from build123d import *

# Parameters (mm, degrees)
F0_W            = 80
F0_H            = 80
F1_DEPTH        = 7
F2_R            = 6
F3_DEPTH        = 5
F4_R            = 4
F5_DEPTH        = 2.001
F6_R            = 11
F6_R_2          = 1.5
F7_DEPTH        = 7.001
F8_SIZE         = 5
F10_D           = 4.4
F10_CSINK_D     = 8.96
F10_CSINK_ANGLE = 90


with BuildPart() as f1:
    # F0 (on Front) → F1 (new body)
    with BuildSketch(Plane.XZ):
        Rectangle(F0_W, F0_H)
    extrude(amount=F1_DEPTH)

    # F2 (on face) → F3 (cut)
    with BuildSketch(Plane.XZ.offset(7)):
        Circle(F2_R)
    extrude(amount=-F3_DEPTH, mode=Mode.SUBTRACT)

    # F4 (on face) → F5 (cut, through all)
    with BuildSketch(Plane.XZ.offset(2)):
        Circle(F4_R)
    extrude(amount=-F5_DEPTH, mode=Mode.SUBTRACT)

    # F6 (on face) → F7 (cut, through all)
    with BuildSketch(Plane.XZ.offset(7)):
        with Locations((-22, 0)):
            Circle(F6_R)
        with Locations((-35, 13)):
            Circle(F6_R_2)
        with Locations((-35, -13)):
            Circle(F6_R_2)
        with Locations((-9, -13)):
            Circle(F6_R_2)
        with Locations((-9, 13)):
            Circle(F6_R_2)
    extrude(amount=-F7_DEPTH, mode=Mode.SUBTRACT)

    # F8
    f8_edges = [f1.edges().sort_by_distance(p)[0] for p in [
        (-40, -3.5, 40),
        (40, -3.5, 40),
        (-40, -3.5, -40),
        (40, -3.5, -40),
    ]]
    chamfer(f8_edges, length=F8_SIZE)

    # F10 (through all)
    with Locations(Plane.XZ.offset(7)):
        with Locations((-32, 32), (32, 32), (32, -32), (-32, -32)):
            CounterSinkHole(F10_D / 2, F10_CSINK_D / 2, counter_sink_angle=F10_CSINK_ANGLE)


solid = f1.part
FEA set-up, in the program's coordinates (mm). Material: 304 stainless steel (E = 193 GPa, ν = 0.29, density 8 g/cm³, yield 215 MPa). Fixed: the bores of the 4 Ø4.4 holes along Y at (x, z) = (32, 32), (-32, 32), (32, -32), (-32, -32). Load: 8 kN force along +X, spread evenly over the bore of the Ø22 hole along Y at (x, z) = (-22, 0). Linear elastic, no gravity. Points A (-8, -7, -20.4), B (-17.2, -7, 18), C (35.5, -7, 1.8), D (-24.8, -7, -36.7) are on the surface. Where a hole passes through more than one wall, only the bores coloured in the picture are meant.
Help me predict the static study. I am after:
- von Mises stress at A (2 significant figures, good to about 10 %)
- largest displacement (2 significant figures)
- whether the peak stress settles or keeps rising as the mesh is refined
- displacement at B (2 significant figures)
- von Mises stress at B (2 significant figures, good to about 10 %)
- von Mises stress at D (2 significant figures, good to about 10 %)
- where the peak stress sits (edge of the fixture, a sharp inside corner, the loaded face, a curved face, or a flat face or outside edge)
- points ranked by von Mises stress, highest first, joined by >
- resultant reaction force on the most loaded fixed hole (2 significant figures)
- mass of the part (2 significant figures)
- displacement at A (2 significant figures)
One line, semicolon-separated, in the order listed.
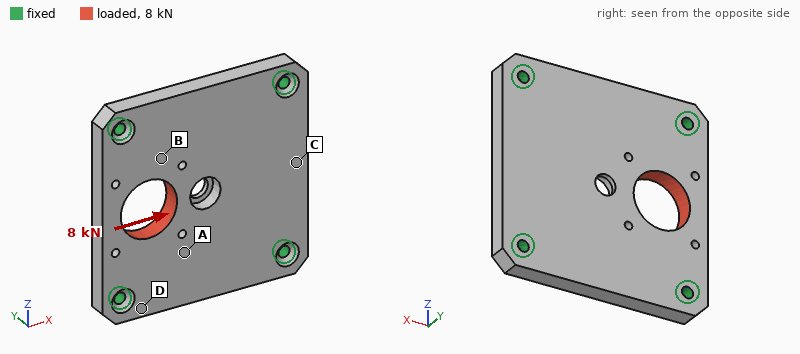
20 MPa; 11 µm; keeps rising; 3.8 µm; 29 MPa; 11 MPa; edge of the fixture; B > A > D > C; 2.3 kN; 320 g; 3.0 µm
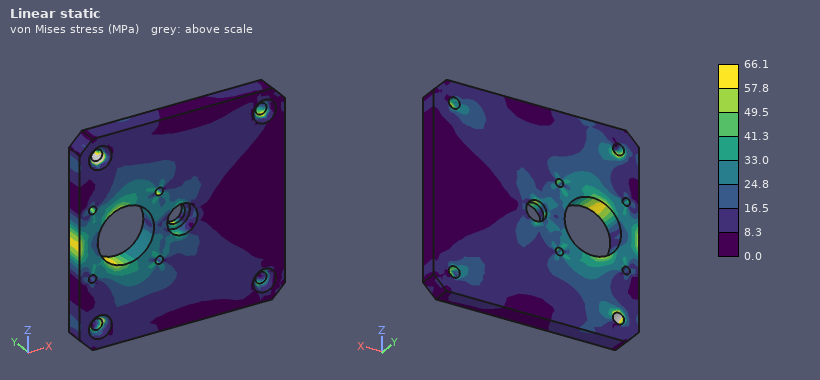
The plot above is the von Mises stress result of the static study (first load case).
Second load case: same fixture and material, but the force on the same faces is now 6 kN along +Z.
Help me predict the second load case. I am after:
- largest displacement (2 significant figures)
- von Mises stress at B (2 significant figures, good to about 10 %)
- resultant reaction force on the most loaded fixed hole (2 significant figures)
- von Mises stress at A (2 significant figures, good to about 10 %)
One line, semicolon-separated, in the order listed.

3.3 µm; 9.5 MPa; 2.3 kN; 5.7 MPa
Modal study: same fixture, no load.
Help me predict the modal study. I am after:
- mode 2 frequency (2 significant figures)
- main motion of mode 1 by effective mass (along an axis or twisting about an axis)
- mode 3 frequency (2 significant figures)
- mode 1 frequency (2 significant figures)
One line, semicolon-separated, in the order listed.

7700 Hz; along Y; 8000 Hz; 4800 Hz
